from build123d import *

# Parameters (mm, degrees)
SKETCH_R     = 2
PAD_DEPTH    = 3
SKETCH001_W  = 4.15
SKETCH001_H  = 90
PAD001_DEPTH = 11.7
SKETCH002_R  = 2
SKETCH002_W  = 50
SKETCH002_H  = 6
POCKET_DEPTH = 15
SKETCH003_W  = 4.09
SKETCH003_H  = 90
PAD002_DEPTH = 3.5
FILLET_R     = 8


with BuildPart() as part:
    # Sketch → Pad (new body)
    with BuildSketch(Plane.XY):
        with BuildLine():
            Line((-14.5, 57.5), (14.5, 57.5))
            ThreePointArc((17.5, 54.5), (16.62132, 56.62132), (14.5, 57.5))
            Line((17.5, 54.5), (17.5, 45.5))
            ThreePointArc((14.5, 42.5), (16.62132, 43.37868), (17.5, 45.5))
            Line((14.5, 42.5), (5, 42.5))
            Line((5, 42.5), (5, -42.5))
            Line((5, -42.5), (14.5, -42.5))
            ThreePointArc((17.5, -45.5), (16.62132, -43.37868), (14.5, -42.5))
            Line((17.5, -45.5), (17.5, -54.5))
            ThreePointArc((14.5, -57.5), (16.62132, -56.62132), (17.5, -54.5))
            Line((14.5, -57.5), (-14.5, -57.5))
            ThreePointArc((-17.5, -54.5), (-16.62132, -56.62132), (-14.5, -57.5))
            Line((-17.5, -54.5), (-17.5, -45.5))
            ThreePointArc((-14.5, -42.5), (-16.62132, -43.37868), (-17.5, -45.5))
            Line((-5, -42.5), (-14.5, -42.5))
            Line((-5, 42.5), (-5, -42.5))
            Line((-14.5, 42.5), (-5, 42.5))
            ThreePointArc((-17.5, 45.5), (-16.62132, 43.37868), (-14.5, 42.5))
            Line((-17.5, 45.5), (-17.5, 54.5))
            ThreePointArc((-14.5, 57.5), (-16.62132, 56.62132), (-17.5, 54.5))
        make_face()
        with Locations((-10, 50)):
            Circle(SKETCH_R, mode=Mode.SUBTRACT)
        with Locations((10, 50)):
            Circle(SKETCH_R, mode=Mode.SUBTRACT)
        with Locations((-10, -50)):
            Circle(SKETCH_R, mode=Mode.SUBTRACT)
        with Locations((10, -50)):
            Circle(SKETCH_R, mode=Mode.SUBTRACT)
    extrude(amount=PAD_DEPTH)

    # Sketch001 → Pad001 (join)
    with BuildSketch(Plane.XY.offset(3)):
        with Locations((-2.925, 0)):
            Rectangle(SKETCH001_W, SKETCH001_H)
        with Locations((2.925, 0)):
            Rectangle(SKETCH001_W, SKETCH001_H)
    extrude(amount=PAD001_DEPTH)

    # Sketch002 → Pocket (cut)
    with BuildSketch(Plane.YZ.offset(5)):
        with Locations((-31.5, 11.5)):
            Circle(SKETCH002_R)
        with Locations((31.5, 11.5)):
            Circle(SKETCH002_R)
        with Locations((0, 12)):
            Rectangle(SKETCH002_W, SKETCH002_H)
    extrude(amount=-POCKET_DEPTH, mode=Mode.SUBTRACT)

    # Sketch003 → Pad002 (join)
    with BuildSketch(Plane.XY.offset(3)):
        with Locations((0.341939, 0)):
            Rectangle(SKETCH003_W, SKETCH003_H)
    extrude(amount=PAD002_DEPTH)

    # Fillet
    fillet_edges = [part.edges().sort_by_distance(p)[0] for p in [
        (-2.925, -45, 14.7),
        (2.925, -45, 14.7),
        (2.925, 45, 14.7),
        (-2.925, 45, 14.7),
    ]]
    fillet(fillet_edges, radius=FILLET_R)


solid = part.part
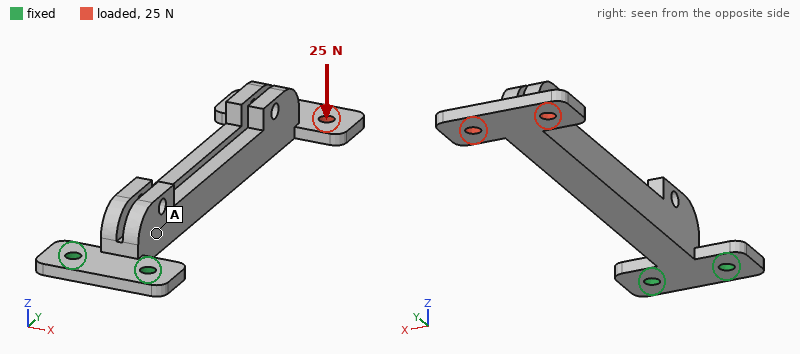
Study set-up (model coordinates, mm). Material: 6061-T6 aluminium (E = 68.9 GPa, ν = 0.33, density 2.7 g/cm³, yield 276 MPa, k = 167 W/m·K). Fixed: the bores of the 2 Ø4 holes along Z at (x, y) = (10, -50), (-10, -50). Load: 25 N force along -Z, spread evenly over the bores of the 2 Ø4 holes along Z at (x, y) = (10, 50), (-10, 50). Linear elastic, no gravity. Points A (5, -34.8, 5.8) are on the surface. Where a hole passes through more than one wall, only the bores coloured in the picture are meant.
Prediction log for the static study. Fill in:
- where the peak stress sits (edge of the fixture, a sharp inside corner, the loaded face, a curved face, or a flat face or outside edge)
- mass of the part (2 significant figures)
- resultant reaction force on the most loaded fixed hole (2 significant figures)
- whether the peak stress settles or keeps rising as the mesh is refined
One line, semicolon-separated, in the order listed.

edge of the fixture; 32 g; 23 N; keeps rising
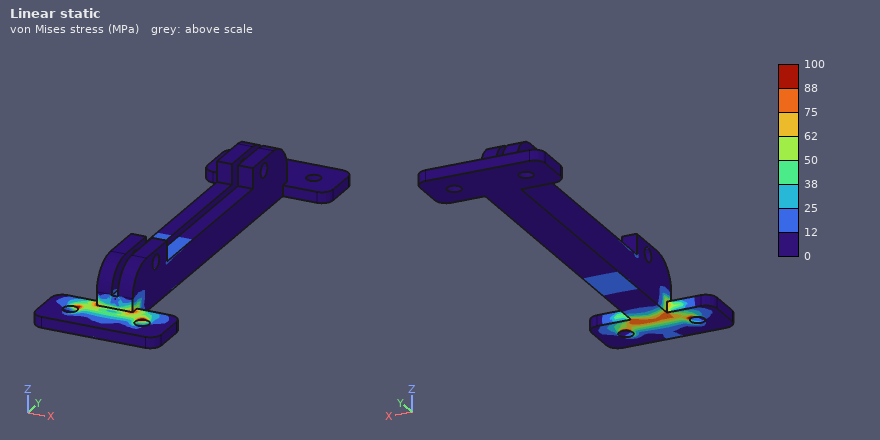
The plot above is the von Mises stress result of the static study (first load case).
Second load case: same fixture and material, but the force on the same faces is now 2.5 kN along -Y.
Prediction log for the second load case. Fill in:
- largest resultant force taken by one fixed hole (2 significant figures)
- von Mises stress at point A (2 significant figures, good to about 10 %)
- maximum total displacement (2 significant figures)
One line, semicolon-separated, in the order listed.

1.3 kN; 17 MPa; 0.86 mm
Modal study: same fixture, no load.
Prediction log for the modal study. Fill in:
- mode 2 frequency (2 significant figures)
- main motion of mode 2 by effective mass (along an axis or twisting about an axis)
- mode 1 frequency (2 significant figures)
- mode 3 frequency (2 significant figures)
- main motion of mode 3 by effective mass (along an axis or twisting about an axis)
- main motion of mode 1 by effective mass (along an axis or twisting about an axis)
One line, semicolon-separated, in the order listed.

600 Hz; along X; 280 Hz; 2700 Hz; twisting about Y; along Z
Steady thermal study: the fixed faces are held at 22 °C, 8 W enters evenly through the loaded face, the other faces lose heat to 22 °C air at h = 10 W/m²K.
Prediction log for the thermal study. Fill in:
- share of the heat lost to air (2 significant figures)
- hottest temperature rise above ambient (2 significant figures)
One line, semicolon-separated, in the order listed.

23 %; 53 K
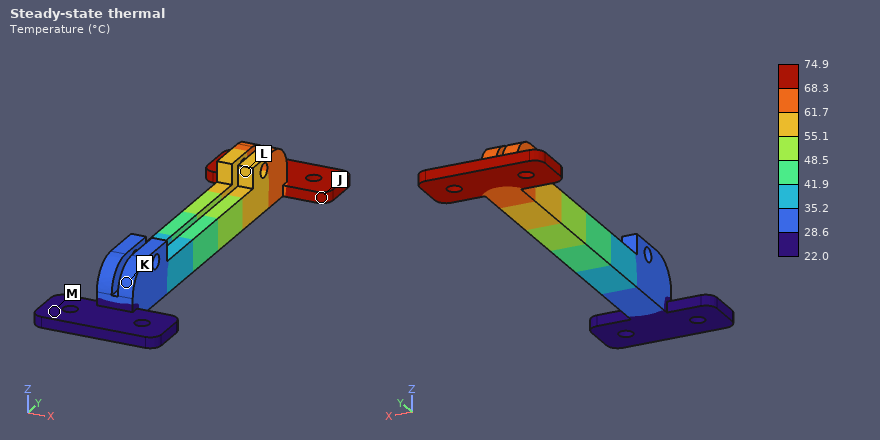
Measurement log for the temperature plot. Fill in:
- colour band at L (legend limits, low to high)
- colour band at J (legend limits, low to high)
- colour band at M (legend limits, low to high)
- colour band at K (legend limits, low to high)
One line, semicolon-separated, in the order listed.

55.1 to 61.7 °C; 68.3 to 74.9 °C; 22.0 to 28.6 °C; 28.6 to 35.2 °C
